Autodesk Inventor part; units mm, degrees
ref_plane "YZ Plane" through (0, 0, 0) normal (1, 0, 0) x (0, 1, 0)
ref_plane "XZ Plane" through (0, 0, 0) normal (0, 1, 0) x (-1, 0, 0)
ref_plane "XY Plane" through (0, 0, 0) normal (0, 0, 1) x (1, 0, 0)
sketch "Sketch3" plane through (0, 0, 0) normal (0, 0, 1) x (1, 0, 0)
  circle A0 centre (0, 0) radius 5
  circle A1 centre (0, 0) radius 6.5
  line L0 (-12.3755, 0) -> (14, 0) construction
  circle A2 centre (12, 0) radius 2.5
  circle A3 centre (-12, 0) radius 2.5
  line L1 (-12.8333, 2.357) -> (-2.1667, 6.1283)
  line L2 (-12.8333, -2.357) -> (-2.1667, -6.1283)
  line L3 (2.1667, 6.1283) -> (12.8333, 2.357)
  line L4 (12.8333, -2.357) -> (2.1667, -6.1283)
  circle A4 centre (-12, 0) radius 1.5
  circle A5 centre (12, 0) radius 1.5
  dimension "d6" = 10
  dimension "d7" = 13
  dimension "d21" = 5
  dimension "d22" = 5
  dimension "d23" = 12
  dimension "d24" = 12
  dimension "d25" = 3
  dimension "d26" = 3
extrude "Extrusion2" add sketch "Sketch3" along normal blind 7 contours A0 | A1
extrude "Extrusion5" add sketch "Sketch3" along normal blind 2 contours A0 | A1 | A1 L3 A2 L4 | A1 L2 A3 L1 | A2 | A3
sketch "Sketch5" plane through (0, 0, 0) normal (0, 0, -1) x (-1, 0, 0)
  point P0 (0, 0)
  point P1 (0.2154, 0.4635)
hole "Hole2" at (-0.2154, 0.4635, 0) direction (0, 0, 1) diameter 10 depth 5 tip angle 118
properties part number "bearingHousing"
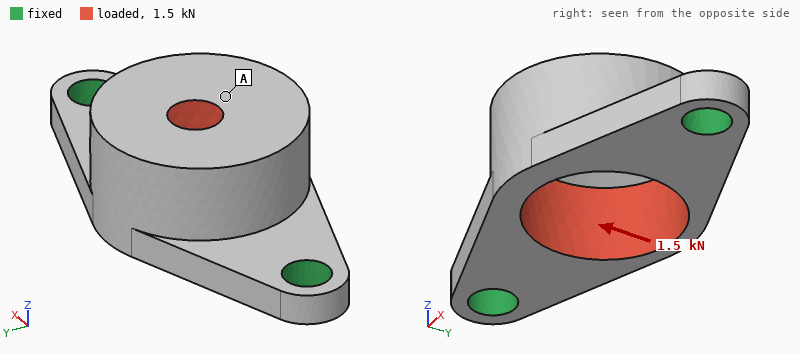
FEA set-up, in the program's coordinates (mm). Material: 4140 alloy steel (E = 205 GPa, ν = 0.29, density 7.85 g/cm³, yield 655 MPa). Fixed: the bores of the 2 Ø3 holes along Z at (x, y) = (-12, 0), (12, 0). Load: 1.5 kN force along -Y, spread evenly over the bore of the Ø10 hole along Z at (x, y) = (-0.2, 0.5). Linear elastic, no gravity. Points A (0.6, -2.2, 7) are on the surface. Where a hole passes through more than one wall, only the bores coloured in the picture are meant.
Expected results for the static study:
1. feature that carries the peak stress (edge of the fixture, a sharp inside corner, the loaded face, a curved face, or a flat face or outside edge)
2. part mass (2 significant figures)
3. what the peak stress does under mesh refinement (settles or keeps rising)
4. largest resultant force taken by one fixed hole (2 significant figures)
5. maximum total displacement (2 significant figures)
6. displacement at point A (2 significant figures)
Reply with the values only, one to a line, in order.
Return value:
edge of the fixture
5.2 g
keeps rising
770 N
42 µm
33 µm
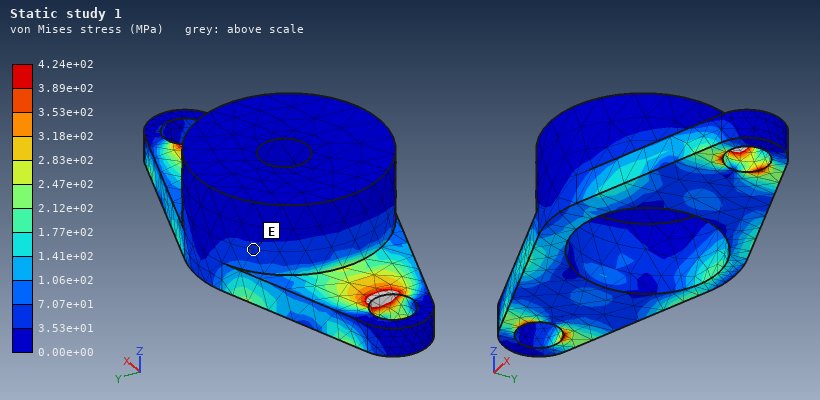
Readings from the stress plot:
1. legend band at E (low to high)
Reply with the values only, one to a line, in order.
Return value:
3.53e+01 to 7.07e+01 MPa
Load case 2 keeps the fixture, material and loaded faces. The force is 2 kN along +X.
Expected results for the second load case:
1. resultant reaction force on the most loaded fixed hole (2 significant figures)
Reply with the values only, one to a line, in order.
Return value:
1.0 kN
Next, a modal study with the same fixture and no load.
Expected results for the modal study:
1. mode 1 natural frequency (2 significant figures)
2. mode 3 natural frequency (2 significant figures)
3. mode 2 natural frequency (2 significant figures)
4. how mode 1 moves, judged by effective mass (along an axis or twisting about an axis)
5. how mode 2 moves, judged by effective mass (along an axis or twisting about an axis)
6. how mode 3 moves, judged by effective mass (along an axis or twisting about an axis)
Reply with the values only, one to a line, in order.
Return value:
11 kHz
33 kHz
21 kHz
along Y
along Z
along X
